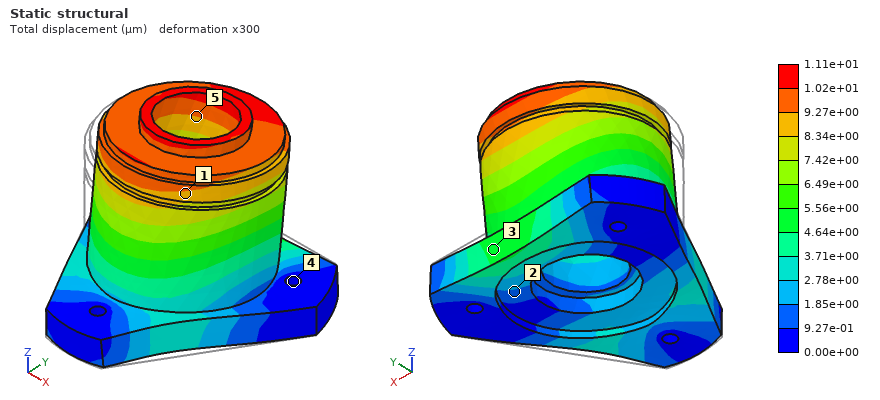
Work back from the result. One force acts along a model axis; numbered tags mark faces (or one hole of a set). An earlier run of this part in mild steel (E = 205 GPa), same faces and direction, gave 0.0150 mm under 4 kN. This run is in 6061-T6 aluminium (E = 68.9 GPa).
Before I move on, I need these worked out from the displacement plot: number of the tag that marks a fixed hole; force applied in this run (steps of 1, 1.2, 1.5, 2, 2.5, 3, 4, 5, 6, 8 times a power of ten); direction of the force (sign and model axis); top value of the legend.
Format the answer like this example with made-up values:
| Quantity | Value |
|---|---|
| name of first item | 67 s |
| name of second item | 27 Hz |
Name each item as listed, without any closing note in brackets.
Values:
| Quantity | Value |
|---|---|
| number of the tag that marks a fixed hole | 4 |
| force applied in this run | 1 kN |
| direction of the force | +Y |
| top value of the legend | 1.11e+01 µm |
